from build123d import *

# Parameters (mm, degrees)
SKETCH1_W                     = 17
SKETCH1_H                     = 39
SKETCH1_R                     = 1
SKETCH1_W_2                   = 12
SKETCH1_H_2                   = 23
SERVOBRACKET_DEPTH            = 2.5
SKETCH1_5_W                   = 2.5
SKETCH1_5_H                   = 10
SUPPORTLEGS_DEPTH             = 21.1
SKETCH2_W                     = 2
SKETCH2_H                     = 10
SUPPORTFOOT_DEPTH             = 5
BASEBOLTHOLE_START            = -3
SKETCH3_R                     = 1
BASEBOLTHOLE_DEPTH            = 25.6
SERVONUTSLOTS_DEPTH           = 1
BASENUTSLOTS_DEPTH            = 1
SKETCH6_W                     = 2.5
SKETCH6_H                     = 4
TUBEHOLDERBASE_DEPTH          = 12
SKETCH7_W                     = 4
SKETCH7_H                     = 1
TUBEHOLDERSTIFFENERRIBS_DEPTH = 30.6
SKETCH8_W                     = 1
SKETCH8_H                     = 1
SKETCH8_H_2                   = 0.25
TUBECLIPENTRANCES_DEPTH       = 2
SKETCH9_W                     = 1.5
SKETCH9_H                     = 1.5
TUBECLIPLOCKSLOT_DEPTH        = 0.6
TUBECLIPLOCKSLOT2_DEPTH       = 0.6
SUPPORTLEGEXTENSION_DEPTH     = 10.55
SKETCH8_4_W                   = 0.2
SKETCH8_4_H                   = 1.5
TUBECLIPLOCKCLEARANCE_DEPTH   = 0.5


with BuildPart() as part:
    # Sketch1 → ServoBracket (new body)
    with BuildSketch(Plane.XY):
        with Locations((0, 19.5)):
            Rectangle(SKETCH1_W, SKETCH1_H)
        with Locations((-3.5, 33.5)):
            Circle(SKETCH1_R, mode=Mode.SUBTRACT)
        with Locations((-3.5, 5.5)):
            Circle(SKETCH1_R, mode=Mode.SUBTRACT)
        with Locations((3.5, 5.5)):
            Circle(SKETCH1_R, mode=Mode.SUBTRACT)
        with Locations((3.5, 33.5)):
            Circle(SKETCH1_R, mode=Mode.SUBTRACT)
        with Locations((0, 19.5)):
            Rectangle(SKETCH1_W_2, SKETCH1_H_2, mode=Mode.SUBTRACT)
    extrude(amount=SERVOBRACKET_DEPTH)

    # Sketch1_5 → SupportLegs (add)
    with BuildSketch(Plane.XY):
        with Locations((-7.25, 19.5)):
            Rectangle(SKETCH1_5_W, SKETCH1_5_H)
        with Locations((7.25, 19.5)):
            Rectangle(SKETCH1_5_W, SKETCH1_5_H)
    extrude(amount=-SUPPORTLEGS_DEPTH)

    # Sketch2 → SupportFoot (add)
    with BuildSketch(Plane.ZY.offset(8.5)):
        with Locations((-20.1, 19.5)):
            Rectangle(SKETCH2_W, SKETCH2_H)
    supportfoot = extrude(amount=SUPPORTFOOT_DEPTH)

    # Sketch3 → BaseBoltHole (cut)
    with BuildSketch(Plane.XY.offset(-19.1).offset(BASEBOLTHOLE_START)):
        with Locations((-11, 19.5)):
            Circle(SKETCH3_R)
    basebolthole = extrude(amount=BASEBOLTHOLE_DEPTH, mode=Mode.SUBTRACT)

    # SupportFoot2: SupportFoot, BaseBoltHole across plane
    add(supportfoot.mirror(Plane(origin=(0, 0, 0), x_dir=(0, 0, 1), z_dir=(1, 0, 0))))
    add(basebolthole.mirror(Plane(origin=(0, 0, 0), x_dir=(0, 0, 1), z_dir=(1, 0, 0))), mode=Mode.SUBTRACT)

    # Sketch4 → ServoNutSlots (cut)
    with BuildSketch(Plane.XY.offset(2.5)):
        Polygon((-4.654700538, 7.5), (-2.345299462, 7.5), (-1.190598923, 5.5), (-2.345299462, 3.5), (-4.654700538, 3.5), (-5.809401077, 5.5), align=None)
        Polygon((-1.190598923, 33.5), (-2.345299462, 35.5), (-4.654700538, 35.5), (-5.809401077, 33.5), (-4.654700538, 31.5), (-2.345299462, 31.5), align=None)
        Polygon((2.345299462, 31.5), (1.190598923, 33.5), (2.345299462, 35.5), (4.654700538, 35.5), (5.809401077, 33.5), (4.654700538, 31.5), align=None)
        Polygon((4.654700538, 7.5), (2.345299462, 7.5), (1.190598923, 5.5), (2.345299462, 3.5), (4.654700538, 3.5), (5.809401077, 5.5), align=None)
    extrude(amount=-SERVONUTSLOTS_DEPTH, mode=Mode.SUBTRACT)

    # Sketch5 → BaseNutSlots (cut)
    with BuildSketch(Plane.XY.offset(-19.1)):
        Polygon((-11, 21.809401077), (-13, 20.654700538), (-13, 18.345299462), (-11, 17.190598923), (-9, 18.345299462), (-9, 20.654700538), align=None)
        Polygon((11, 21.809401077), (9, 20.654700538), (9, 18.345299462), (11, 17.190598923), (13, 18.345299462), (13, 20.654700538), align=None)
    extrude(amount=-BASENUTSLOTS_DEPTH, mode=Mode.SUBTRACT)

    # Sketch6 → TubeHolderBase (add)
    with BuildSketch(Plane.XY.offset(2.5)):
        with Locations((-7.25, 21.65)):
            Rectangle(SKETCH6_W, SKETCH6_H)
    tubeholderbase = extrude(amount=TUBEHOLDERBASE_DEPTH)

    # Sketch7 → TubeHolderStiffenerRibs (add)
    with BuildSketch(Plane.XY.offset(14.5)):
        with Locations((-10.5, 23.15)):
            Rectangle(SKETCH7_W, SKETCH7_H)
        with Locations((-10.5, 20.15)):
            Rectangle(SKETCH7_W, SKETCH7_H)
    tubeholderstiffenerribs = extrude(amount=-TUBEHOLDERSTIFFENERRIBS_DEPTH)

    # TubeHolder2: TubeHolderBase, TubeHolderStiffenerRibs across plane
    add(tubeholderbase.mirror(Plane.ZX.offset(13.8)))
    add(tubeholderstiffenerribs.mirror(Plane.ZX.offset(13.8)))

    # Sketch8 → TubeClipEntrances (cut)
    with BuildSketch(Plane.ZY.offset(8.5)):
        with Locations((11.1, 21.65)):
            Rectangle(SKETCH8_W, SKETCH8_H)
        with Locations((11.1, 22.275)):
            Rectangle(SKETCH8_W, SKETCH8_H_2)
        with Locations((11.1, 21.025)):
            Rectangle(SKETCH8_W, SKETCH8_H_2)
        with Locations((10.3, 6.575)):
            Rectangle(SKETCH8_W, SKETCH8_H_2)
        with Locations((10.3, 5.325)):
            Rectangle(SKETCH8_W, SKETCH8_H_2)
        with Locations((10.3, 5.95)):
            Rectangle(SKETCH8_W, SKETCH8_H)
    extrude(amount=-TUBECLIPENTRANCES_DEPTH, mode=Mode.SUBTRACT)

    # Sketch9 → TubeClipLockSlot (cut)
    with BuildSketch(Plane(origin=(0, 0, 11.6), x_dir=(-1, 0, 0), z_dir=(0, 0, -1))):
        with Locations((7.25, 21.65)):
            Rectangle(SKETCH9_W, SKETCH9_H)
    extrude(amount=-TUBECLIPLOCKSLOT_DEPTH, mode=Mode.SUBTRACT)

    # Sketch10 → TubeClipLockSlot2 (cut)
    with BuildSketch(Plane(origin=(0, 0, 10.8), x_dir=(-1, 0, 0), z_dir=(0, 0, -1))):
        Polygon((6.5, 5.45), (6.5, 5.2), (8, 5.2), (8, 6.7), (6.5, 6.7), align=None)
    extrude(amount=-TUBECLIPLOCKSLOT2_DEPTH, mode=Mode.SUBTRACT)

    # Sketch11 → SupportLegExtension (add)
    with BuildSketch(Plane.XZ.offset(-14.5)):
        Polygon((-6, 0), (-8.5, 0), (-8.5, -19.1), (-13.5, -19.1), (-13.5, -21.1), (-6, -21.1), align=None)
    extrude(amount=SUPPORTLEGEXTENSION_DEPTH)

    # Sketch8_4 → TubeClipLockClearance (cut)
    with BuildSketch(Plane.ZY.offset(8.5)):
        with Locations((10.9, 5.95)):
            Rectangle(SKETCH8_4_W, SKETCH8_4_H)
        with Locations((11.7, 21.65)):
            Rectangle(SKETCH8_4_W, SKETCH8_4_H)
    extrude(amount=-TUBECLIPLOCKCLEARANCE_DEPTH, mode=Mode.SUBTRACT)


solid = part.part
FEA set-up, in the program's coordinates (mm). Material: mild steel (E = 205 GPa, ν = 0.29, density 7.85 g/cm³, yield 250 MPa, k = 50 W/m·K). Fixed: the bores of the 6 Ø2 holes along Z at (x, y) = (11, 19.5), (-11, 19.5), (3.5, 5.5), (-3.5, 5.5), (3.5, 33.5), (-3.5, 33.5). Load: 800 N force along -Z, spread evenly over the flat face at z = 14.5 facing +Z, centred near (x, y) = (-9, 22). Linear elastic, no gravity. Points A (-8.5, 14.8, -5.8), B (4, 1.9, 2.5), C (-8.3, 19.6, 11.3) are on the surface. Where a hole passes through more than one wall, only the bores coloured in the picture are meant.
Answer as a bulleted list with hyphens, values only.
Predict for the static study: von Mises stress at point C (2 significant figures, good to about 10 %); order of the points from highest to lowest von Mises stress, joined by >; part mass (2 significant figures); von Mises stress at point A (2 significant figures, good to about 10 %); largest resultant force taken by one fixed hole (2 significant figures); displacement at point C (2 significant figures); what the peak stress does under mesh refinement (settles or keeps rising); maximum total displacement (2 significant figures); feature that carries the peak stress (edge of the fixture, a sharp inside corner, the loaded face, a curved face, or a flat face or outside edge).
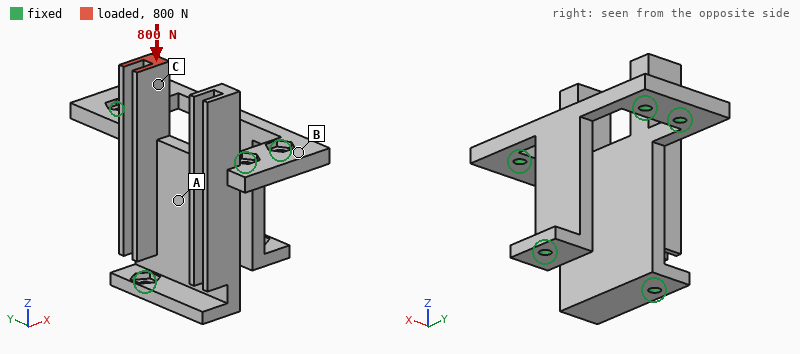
- 49 MPa
- C > A > B
- 27 g
- 31 MPa
- 480 N
- 14 µm
- keeps rising
- 20 µm
- edge of the fixture
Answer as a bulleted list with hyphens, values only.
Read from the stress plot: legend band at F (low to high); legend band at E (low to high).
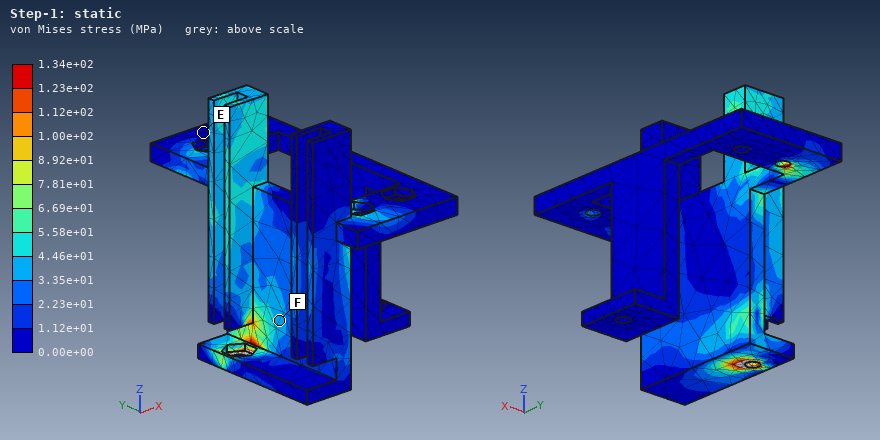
- 3.35e+01 to 4.46e+01 MPa
- 0.00e+00 to 1.12e+01 MPa
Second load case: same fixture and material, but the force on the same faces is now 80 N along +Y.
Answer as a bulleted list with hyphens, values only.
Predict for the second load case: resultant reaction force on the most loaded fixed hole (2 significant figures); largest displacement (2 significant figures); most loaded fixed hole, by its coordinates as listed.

- 81 N
- 29 µm
- (-3.5, 33.5)
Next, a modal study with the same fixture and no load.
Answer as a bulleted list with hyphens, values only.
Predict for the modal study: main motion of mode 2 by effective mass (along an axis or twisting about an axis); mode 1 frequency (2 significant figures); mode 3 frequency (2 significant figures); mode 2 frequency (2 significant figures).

- along X
- 7800 Hz
- 10 kHz
- 8300 Hz
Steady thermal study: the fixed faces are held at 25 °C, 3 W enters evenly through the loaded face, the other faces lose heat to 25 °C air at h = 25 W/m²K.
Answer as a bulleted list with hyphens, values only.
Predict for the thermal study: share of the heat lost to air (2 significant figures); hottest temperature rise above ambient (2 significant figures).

- 28 %
- 62 K
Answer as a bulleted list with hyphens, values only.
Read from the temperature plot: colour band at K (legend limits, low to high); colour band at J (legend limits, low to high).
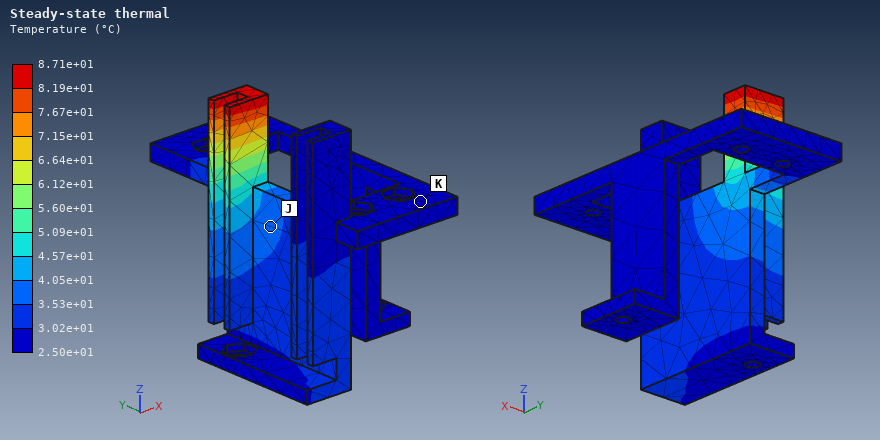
- 2.50e+01 to 3.02e+01 °C
- 3.53e+01 to 4.05e+01 °C
